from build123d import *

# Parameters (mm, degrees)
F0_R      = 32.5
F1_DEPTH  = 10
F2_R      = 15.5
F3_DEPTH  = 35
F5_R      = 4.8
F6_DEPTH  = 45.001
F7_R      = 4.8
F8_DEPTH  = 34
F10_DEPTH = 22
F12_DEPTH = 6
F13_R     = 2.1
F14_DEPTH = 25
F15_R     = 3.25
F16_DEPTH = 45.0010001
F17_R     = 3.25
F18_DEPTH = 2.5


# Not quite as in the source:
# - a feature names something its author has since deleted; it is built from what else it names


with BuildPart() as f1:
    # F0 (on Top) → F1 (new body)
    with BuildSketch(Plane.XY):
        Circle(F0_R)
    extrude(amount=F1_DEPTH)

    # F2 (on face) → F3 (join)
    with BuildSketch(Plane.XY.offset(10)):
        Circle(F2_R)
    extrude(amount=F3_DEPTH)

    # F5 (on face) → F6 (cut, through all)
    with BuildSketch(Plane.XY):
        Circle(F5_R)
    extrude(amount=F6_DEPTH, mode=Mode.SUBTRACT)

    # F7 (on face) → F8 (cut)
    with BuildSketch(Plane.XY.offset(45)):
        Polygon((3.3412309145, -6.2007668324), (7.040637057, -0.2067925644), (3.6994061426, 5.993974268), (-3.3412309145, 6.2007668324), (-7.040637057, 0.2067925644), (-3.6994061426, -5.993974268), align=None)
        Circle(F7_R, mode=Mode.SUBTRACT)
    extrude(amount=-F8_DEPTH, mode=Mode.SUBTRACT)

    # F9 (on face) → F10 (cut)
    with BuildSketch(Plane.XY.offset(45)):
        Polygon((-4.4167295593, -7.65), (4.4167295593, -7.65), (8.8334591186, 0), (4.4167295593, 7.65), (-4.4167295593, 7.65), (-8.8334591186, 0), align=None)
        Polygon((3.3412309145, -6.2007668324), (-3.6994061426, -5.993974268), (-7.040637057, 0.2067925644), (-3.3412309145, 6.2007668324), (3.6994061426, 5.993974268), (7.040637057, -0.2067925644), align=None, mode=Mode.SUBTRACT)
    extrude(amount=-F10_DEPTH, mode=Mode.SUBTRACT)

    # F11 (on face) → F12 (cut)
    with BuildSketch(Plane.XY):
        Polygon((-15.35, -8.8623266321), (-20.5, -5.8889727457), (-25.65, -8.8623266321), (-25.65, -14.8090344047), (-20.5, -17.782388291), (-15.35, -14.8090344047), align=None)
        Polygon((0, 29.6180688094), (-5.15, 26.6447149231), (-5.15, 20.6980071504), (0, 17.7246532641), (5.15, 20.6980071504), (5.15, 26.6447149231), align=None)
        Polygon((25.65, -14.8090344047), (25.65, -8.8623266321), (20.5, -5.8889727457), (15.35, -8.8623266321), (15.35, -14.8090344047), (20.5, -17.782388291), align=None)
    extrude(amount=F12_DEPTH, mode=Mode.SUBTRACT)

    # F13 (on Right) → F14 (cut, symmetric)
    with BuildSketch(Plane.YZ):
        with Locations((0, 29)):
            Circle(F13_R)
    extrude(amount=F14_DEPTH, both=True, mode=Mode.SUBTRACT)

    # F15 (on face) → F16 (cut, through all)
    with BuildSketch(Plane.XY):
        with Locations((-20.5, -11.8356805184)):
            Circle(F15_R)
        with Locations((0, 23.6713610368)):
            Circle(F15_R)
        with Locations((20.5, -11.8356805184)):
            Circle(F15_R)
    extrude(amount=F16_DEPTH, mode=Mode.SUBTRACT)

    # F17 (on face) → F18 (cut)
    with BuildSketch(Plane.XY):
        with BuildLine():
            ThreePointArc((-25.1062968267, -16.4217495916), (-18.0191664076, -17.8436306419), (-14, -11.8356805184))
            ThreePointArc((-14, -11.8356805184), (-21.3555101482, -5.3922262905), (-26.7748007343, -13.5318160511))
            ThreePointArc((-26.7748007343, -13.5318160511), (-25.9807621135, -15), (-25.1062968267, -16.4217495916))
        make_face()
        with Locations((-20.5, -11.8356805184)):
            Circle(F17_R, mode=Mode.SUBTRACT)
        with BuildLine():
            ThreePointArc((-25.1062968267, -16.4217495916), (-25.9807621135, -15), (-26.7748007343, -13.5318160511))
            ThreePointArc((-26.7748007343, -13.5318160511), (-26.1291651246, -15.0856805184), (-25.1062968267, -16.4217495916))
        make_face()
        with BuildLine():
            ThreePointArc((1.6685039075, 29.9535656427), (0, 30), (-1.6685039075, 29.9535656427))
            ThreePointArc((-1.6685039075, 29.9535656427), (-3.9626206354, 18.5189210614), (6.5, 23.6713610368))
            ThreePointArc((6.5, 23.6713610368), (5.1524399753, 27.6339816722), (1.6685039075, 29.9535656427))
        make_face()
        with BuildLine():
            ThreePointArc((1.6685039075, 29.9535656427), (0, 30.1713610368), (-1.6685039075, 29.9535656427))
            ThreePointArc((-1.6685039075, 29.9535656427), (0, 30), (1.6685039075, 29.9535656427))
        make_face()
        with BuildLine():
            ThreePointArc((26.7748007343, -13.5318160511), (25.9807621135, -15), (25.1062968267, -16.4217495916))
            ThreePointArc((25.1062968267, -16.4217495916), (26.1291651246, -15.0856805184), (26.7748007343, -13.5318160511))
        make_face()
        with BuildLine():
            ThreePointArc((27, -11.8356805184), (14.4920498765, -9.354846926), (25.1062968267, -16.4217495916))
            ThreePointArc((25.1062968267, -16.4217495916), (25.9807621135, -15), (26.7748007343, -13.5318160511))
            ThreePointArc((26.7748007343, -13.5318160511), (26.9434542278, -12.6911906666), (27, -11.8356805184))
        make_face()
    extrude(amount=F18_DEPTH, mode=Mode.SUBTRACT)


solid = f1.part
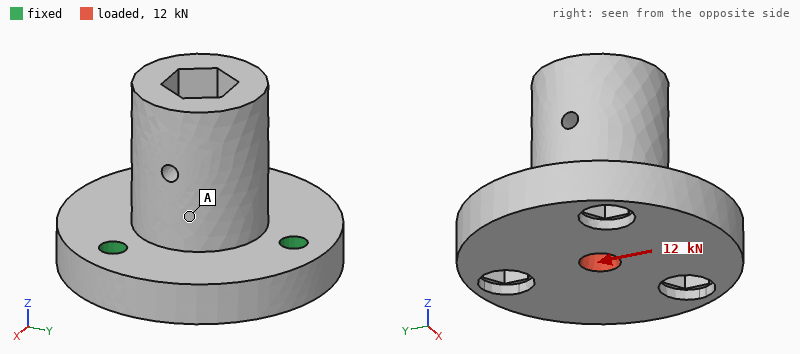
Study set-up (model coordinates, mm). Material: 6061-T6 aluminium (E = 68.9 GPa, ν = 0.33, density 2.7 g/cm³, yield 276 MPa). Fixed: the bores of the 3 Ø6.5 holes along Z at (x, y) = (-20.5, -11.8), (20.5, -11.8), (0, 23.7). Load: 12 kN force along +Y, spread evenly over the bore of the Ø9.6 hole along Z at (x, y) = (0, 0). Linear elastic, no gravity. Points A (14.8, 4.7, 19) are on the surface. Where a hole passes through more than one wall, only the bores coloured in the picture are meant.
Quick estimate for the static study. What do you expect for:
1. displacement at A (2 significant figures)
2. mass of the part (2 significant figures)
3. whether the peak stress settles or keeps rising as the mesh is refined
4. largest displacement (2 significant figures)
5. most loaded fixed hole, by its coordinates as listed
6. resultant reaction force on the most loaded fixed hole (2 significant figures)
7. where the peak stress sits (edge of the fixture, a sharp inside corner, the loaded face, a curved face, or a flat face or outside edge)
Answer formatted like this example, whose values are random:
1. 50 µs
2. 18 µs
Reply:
1. 6.9 µm
2. 140 g
3. keeps rising
4. 16 µm
5. (0, 23.7)
6. 4.6 kN
7. edge of the fixture
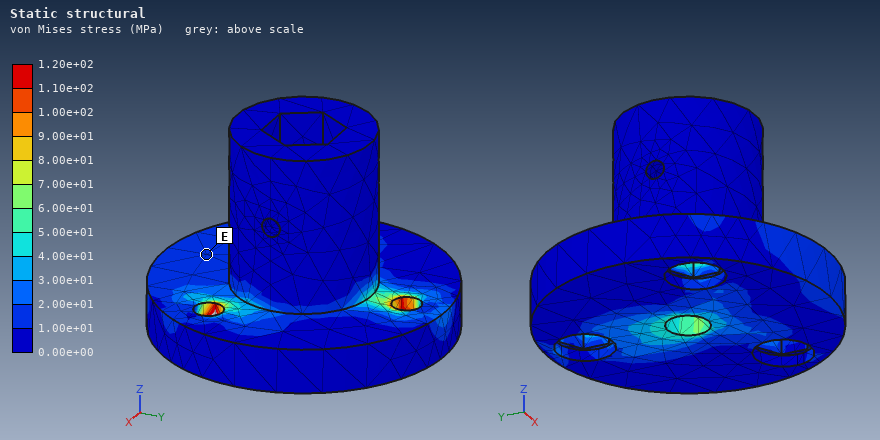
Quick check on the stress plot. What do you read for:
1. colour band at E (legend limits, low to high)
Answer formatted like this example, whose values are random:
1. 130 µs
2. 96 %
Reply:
1. 1.00e+01 to 2.00e+01 MPa
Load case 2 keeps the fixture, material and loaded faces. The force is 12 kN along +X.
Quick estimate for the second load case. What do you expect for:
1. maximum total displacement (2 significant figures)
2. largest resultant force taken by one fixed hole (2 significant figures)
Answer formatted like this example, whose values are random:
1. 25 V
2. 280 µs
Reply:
1. 15 µm
2. 4.3 kN
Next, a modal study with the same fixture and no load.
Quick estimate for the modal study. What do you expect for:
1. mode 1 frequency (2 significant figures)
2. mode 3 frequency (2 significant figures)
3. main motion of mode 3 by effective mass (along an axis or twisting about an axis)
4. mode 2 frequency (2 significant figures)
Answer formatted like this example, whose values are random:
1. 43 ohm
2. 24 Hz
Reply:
1. 7300 Hz
2. 11 kHz
3. along Z
4. 7400 Hz
